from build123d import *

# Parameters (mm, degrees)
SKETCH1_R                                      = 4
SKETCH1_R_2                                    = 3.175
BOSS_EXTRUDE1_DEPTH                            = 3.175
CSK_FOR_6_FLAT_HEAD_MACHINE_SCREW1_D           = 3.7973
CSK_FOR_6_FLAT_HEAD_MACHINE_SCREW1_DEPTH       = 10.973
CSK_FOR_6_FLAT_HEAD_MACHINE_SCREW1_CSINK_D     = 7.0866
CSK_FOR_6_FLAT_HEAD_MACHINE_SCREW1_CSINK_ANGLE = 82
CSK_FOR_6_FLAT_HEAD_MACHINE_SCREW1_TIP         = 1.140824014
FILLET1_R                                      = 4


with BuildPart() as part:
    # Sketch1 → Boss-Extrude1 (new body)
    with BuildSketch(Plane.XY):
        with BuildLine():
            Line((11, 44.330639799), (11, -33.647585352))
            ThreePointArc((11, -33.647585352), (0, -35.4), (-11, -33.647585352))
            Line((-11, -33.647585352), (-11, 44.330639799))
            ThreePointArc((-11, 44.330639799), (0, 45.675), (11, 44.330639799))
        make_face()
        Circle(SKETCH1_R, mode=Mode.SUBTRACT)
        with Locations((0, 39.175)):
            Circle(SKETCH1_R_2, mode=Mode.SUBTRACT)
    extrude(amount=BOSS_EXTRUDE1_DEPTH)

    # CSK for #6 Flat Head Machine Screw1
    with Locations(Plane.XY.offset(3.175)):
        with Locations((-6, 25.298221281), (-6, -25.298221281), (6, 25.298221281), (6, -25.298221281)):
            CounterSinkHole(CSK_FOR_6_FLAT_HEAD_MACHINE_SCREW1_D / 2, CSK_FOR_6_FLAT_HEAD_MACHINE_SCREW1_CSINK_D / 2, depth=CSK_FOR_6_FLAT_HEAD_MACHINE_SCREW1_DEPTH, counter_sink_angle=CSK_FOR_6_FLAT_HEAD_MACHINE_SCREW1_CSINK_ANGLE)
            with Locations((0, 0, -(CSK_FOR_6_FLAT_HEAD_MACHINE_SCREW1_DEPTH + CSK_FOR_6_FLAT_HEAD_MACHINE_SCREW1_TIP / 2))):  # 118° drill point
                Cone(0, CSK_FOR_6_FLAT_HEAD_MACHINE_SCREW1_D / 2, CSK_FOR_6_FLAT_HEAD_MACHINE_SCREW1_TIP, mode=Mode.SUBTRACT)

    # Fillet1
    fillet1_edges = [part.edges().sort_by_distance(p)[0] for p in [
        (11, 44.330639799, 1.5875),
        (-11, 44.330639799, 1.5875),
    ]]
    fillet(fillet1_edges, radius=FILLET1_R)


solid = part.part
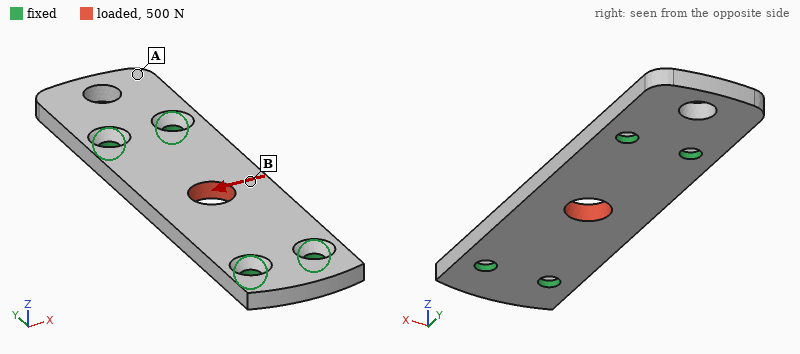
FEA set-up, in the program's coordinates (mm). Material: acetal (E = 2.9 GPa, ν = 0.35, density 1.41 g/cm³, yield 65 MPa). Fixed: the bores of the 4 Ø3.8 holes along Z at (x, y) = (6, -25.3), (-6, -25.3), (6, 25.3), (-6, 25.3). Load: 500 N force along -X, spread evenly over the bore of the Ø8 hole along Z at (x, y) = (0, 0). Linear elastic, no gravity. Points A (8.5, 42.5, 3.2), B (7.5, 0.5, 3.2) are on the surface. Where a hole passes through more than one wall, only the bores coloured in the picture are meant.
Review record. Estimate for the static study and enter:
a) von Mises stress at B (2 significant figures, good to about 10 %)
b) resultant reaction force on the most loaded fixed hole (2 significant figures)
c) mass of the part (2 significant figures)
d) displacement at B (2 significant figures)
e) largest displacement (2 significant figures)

8.8 MPa
220 N
7.2 g
0.14 mm
0.16 mm
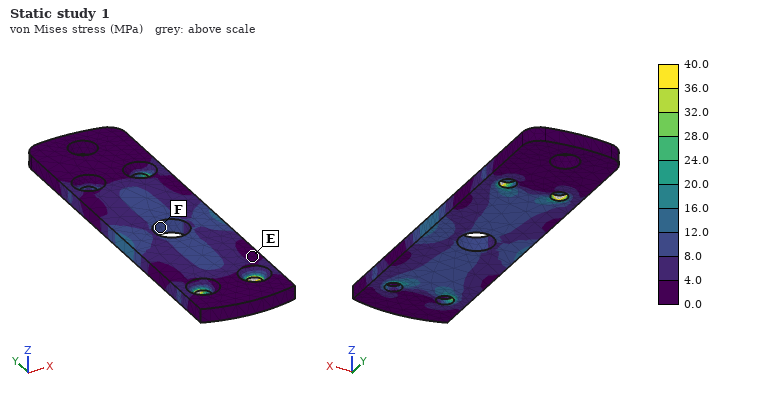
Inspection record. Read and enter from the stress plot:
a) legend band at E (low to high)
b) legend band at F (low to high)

0.0 to 4.0 MPa
8.0 to 12.0 MPa
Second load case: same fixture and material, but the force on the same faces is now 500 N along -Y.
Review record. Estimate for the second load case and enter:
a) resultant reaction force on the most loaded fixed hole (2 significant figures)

130 N
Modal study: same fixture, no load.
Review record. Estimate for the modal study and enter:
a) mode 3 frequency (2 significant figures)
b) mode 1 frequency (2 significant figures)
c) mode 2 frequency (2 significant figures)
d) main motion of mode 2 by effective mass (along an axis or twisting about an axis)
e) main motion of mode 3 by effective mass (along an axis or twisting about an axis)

2800 Hz
1500 Hz
1700 Hz
along Z
twisting about Y
